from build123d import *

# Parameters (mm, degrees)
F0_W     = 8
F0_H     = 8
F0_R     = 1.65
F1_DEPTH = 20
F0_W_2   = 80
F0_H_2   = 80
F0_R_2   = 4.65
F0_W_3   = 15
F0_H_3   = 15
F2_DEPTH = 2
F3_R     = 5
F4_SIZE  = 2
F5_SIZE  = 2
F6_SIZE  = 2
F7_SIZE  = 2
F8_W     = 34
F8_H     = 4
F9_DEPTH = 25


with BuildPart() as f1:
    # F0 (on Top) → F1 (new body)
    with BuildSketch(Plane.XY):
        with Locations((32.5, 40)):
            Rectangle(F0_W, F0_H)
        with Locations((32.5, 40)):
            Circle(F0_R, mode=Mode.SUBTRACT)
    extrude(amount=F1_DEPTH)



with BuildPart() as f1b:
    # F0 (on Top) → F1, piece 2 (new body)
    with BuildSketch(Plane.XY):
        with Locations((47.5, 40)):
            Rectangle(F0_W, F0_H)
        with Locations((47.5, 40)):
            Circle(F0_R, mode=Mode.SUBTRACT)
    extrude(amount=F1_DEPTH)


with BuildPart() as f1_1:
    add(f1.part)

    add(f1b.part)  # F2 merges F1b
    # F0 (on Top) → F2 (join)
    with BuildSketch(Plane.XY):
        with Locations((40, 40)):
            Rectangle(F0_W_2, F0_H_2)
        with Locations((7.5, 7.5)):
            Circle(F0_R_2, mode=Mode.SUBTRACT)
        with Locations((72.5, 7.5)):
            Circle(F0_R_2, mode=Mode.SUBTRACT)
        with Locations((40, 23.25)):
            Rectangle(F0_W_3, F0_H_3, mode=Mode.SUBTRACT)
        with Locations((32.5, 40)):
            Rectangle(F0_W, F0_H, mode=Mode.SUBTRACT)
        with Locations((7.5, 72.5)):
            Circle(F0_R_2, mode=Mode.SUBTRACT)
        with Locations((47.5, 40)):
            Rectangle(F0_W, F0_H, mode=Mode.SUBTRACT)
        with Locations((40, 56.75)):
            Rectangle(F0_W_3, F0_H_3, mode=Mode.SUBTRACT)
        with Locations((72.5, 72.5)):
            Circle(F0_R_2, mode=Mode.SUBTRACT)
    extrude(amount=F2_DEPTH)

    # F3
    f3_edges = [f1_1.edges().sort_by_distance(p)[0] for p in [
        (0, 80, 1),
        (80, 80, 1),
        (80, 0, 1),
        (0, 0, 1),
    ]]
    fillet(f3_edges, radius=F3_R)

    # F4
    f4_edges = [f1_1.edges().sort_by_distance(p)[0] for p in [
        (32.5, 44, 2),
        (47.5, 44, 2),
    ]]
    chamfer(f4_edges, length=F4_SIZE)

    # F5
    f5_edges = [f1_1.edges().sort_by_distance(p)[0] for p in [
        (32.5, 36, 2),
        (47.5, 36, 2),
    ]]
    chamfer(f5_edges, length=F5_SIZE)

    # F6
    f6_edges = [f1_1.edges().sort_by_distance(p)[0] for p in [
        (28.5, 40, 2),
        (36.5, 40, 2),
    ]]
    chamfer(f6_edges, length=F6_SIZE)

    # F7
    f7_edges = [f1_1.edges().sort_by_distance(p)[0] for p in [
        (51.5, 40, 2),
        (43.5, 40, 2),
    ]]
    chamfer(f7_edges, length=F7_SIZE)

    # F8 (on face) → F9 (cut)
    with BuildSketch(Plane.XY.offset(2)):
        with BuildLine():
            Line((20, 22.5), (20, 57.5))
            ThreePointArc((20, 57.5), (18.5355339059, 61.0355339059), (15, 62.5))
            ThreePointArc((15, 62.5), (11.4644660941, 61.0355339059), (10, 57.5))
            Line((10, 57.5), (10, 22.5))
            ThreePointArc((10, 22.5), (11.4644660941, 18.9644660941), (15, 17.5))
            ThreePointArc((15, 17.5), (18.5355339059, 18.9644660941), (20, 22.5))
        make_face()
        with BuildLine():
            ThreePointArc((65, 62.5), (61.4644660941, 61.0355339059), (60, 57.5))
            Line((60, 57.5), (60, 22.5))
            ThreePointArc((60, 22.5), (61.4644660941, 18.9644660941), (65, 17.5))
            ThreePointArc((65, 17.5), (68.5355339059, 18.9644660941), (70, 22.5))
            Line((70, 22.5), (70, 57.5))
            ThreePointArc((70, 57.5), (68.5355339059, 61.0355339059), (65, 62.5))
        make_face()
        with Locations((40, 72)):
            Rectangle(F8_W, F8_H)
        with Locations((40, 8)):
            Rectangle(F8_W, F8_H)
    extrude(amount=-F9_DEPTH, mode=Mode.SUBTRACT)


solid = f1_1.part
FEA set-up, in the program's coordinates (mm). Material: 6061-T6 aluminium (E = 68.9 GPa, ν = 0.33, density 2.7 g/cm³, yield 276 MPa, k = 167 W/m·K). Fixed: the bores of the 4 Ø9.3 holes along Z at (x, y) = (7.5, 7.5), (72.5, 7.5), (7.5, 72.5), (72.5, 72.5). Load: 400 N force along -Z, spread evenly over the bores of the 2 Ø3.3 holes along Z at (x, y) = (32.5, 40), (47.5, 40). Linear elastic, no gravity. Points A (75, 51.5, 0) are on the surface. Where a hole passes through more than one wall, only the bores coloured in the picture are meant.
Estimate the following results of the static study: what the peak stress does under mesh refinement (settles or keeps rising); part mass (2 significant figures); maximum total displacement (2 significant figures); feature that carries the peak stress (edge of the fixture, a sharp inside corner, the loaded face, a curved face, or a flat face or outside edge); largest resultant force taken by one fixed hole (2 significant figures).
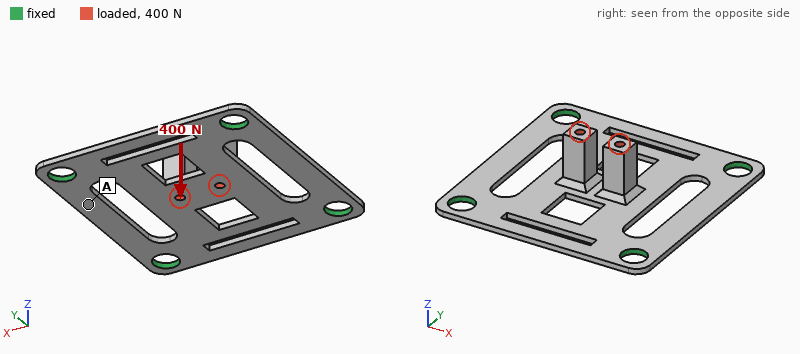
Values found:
keeps rising
30 g
0.50 mm
a sharp inside corner
110 N
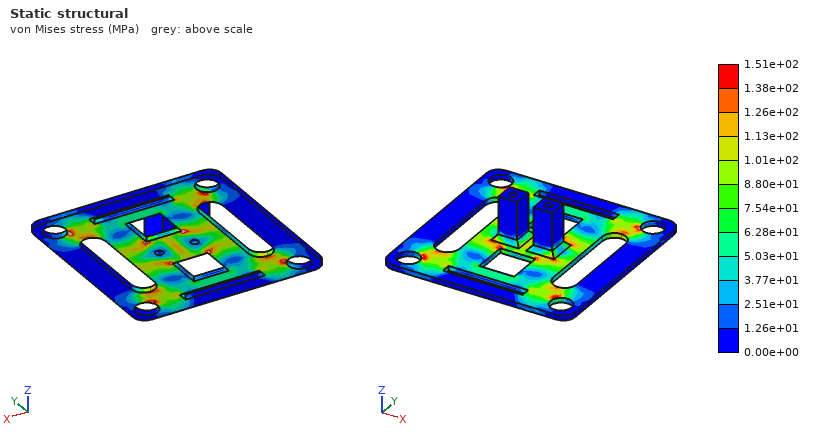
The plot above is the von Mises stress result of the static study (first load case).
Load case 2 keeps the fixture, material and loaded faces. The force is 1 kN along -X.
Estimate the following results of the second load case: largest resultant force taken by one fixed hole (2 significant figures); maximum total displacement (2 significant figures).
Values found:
340 N
0.50 mm
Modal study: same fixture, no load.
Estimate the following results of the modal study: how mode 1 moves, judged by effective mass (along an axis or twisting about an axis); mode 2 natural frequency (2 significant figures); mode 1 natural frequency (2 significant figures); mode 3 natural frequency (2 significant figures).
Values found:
along Z
2400 Hz
1400 Hz
2800 Hz
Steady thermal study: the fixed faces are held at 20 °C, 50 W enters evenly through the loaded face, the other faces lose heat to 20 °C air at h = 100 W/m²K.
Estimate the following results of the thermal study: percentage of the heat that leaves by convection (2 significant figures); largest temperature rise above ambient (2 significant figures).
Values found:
53 %
78 K
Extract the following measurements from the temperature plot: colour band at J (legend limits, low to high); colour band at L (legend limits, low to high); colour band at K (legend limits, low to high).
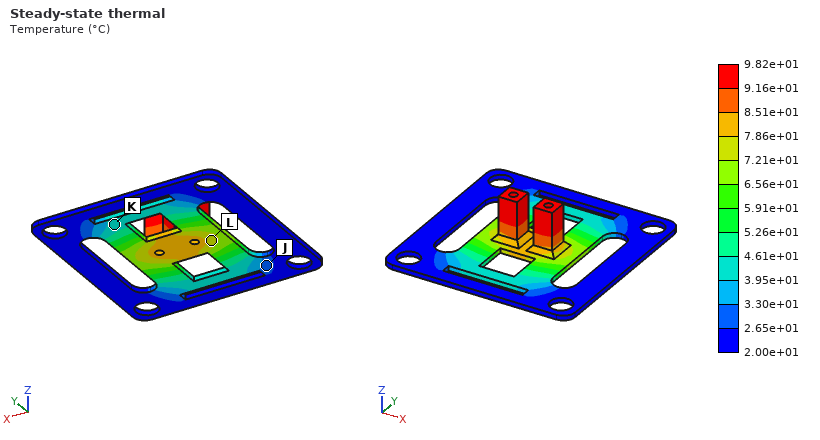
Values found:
2.65e+01 to 3.30e+01 °C
7.21e+01 to 7.86e+01 °C
3.95e+01 to 4.61e+01 °C
